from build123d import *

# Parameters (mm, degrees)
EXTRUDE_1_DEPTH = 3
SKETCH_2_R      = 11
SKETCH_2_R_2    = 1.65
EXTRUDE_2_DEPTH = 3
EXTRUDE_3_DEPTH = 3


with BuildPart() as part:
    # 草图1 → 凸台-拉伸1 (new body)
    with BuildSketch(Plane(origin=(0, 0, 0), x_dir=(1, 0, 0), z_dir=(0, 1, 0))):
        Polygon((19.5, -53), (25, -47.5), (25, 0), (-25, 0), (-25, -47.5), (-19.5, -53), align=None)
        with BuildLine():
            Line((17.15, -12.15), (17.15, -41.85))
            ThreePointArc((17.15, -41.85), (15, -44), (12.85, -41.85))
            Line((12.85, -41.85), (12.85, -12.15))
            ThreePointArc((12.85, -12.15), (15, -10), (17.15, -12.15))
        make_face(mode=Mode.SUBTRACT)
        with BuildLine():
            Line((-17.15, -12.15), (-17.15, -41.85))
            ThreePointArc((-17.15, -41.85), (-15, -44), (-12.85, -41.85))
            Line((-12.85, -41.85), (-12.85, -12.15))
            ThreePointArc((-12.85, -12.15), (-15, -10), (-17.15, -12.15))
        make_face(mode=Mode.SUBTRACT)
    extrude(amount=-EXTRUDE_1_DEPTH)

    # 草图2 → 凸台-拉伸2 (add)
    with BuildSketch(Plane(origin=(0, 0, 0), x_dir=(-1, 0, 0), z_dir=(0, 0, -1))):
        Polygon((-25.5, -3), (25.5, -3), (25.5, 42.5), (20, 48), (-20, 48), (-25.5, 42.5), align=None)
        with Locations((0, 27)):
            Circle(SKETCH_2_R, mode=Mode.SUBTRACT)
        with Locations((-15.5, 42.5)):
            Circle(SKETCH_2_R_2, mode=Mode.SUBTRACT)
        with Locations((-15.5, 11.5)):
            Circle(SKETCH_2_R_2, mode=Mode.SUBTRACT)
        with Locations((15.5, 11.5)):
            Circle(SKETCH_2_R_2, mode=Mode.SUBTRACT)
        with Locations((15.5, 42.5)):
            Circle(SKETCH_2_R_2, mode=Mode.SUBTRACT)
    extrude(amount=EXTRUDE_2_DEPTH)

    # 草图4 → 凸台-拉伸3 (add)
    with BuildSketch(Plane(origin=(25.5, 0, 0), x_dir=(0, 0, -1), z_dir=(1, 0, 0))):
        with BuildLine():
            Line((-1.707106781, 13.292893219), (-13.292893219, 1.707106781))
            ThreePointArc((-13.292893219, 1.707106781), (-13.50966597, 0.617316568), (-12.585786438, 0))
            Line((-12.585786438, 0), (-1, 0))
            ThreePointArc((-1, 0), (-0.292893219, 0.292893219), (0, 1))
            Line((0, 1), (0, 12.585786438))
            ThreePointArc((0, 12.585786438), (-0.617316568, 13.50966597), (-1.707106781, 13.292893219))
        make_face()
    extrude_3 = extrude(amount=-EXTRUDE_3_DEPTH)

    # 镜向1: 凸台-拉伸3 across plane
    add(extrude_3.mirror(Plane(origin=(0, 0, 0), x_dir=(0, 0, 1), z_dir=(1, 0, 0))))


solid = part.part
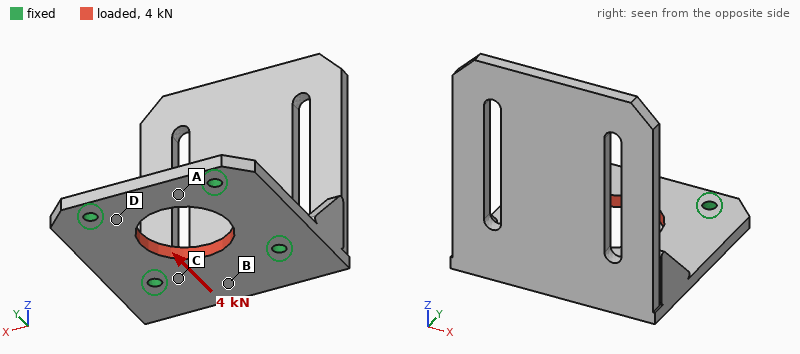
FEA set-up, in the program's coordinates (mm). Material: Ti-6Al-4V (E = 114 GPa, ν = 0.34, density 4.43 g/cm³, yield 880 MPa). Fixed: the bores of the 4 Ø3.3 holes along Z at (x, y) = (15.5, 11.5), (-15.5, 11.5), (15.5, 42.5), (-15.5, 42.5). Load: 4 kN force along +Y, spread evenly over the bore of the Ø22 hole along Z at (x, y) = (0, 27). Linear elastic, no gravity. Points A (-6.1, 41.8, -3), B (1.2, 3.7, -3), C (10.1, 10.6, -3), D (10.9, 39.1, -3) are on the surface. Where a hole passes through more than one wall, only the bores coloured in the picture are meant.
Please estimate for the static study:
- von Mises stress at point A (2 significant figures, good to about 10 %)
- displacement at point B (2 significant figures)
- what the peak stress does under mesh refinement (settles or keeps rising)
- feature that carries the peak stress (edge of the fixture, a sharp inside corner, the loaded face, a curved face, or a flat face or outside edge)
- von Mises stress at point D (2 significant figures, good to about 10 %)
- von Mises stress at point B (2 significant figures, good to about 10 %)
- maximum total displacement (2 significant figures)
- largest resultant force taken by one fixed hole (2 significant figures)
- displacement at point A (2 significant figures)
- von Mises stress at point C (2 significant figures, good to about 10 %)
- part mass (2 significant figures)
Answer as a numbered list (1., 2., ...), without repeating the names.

1. 25 MPa
2. 2.9 µm
3. keeps rising
4. edge of the fixture
5. 30 MPa
6. 8.7 MPa
7. 7.5 µm
8. 1.0 kN
9. 5.3 µm
10. 16 MPa
11. 63 g
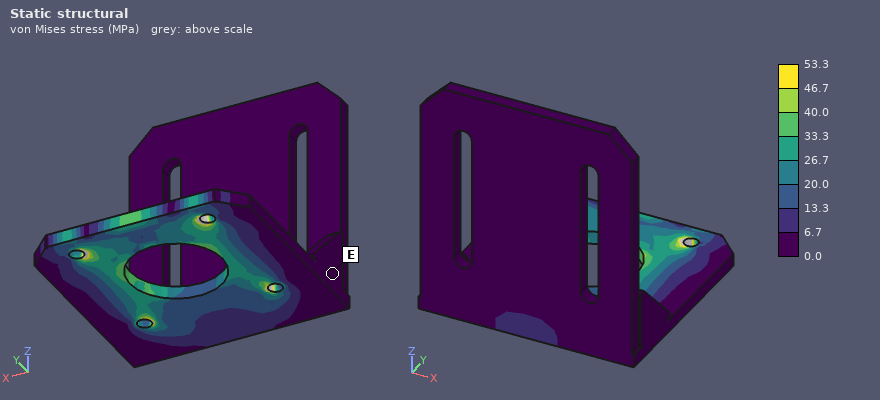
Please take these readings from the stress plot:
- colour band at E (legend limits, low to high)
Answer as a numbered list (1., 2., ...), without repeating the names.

1. 0.0 to 6.7 MPa
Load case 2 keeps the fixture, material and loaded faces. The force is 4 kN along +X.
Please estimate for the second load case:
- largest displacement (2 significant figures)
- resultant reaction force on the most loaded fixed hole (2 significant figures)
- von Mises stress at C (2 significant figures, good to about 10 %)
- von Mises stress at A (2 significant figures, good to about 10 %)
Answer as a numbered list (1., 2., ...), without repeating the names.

1. 5.6 µm
2. 1.0 kN
3. 21 MPa
4. 22 MPa
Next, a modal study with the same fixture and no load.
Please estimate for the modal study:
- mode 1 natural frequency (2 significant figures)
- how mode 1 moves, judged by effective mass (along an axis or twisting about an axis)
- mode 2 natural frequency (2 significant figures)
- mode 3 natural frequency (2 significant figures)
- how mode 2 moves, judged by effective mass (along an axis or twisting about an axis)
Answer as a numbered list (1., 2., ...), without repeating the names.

1. 800 Hz
2. along Y
3. 1900 Hz
4. 3000 Hz
5. along X
